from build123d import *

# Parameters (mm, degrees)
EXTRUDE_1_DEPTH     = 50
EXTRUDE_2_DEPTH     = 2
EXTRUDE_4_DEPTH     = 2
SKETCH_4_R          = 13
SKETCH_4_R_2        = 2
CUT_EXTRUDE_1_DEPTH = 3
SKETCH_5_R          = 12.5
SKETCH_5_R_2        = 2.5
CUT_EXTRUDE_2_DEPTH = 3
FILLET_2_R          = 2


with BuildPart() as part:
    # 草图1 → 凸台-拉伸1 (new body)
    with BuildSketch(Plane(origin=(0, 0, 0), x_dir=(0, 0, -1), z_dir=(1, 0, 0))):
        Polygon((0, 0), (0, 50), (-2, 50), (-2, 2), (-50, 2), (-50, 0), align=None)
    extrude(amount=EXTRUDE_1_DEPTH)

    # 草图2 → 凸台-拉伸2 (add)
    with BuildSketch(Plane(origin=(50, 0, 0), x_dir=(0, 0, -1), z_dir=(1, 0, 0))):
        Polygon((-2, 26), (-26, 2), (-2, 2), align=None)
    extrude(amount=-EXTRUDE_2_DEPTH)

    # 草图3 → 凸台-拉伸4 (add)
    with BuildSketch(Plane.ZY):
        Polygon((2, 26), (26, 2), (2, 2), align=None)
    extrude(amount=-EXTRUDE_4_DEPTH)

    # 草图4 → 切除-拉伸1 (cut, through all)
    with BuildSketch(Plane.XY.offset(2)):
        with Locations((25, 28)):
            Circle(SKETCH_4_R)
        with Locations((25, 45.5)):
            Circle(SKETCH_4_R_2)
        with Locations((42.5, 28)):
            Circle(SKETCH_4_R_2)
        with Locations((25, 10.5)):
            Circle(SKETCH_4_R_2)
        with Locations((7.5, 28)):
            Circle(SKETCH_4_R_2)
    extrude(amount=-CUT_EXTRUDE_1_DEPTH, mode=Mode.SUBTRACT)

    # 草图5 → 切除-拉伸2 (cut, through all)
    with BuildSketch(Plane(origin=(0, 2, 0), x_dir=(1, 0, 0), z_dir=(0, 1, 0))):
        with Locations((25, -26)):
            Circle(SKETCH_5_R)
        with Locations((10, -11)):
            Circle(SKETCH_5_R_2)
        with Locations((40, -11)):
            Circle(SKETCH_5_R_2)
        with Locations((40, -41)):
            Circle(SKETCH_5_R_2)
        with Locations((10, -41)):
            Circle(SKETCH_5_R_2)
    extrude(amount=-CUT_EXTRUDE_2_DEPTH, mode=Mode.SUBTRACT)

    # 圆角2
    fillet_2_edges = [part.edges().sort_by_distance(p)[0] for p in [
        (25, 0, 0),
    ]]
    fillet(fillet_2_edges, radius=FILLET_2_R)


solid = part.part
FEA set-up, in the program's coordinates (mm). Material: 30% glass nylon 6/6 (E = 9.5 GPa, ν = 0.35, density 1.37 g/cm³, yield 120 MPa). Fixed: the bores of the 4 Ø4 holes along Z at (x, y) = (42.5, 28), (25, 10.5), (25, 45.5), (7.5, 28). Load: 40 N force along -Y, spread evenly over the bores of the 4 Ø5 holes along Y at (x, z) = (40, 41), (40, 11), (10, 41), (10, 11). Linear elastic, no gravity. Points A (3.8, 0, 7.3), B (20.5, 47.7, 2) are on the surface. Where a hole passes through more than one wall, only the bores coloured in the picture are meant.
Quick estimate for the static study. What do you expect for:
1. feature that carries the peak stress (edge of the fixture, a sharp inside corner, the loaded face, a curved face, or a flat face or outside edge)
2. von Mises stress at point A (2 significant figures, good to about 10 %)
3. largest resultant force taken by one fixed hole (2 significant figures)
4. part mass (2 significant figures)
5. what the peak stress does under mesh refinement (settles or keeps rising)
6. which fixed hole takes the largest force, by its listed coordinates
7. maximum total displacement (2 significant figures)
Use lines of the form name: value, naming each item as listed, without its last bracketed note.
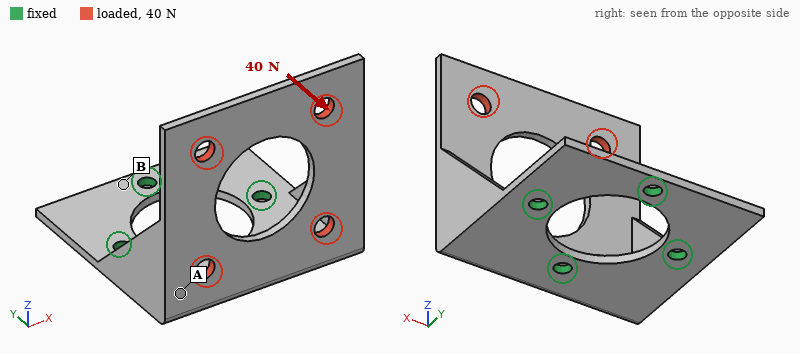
feature that carries the peak stress: edge of the fixture
von Mises stress at point A: 5.1 MPa
largest resultant force taken by one fixed hole: 44 N
part mass: 12 g
what the peak stress does under mesh refinement: keeps rising
which fixed hole takes the largest force, by its listed coordinates: (25, 10.5)
maximum total displacement: 0.89 mm
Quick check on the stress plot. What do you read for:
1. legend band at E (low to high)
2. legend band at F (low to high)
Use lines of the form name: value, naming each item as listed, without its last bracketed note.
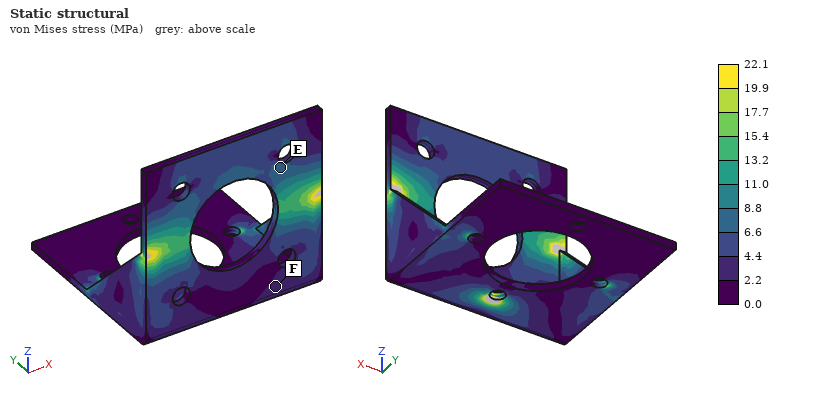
legend band at E: 6.6 to 8.8 MPa
legend band at F: 2.2 to 4.4 MPa
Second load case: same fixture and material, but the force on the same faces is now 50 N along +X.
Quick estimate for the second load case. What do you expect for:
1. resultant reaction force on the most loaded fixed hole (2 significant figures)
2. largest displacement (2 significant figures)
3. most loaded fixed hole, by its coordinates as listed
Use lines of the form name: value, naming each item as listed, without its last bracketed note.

resultant reaction force on the most loaded fixed hole: 45 N
largest displacement: 0.96 mm
most loaded fixed hole, by its coordinates as listed: (25, 10.5)
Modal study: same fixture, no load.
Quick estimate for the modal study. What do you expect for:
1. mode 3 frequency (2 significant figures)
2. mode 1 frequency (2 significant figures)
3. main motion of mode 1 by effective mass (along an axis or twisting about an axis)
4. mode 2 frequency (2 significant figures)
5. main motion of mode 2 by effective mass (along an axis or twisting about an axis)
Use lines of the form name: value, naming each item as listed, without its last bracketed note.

mode 3 frequency: 1600 Hz
mode 1 frequency: 520 Hz
main motion of mode 1 by effective mass: along X
mode 2 frequency: 600 Hz
main motion of mode 2 by effective mass: along Y
